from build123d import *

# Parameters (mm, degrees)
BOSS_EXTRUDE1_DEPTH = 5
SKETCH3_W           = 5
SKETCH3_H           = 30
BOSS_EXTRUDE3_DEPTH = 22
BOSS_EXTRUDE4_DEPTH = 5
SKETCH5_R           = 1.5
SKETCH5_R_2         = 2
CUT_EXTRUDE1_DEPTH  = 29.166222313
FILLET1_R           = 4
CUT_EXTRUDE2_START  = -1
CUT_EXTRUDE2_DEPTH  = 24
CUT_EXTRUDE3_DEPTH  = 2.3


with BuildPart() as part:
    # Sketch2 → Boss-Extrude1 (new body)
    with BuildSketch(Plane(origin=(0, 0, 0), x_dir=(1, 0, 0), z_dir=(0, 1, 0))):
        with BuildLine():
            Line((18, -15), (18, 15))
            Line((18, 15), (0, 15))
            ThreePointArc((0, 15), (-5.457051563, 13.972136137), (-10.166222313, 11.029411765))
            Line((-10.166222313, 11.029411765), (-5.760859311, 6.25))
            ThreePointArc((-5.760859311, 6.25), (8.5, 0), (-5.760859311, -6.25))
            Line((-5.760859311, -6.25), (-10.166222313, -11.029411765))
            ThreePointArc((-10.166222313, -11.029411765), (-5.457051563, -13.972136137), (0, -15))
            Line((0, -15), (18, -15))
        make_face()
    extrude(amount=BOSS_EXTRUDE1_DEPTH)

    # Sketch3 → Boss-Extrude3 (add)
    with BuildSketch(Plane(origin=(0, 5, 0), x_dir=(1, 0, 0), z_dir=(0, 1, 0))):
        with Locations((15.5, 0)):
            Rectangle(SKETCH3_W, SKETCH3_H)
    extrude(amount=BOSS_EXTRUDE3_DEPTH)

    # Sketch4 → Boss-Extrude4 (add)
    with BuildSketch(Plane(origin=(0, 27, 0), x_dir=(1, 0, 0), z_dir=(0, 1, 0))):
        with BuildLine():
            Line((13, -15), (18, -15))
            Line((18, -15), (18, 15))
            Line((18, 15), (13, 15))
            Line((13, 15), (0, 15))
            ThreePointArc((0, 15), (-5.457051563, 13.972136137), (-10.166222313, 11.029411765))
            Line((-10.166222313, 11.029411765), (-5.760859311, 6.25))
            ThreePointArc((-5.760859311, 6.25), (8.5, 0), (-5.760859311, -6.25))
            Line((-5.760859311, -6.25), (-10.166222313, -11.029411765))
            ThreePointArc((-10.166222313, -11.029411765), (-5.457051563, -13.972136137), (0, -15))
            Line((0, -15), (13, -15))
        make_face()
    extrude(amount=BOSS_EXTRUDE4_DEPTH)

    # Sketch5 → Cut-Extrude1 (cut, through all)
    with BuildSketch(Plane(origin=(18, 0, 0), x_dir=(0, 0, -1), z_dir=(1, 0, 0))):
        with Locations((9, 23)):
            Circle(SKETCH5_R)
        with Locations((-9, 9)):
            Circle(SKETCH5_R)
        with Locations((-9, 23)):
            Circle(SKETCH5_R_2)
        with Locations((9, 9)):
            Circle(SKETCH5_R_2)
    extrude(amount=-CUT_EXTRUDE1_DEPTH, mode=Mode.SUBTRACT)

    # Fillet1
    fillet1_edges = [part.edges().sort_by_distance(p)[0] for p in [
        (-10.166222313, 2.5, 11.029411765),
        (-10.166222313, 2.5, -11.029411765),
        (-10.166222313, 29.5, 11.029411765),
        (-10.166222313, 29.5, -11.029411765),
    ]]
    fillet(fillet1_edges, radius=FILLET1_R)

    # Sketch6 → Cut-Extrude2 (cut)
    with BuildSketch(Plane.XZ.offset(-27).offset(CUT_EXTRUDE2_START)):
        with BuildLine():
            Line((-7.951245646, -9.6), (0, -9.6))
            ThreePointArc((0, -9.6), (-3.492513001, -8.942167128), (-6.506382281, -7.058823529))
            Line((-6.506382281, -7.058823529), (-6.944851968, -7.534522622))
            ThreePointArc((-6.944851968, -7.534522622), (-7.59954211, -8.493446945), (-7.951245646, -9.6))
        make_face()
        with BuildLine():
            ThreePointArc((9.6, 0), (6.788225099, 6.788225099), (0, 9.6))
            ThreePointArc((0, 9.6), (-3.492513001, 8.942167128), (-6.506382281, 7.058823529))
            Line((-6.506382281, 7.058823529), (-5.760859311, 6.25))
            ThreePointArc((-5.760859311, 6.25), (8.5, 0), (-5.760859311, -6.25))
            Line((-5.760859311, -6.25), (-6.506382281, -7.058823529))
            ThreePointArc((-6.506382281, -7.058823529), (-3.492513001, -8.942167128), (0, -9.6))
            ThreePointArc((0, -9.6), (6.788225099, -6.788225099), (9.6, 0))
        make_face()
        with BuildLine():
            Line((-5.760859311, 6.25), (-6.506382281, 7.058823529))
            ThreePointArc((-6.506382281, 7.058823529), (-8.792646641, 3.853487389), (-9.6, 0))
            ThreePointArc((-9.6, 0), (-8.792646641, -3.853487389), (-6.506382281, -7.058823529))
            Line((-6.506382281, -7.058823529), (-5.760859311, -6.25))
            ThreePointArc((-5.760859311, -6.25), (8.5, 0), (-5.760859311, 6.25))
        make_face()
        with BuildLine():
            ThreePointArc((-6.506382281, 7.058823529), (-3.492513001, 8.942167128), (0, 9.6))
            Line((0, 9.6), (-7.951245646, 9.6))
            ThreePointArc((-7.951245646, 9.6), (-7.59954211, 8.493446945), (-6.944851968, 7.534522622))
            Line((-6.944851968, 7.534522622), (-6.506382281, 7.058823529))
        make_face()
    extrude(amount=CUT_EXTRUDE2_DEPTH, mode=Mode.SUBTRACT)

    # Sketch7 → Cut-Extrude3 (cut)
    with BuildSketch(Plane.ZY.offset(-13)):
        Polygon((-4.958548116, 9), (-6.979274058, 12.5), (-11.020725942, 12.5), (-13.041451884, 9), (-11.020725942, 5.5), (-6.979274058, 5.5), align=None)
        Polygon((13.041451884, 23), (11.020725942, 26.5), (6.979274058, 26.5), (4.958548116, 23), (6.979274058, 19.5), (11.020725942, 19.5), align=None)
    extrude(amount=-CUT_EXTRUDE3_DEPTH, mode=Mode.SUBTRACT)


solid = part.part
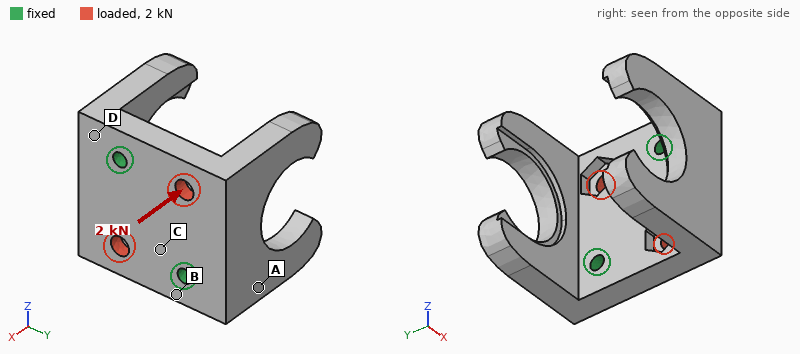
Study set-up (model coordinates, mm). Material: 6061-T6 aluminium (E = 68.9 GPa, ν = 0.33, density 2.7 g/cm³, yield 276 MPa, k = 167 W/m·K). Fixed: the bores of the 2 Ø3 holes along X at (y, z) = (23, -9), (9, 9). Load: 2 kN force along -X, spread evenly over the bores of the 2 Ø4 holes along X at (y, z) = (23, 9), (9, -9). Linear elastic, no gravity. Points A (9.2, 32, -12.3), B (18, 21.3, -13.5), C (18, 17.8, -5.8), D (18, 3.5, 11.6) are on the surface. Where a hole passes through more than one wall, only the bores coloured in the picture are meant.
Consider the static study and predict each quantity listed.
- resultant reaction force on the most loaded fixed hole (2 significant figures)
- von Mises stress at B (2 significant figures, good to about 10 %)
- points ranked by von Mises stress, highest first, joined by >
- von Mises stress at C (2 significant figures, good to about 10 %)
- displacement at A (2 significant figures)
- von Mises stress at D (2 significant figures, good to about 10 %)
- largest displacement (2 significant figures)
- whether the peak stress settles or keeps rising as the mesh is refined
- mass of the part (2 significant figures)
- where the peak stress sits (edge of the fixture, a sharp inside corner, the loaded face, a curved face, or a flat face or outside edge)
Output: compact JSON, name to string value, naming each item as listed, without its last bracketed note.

{"resultant reaction force on the most loaded fixed hole": "1.0 kN", "von Mises stress at B": "46 MPa", "points ranked by von Mises stress, highest first, joined by >": "C > B > D > A", "von Mises stress at C": "64 MPa", "displacement at A": "12 µm", "von Mises stress at D": "25 MPa", "largest displacement": "75 µm", "whether the peak stress settles or keeps rising as the mesh is refined": "keeps rising", "mass of the part": "22 g", "where the peak stress sits": "edge of the fixture"}
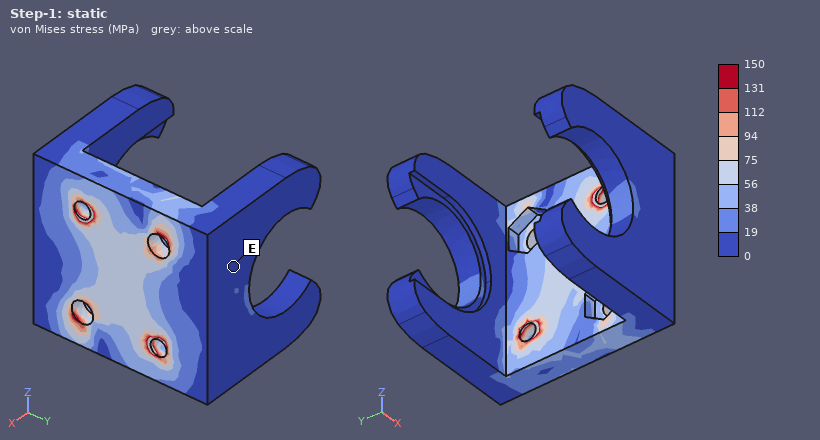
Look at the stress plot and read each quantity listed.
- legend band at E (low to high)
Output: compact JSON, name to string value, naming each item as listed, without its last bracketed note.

{"legend band at E": "0 to 19 MPa"}
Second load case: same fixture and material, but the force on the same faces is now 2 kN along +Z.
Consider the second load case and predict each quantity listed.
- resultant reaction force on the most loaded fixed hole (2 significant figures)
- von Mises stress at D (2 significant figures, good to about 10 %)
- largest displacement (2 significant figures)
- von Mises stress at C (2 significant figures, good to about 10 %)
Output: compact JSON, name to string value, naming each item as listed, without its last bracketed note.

{"resultant reaction force on the most loaded fixed hole": "1.0 kN", "von Mises stress at D": "6.9 MPa", "largest displacement": "12 µm", "von Mises stress at C": "13 MPa"}
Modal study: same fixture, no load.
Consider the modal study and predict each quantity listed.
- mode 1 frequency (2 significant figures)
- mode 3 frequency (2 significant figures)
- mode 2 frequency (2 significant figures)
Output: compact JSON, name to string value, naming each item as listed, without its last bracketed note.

{"mode 1 frequency": "5200 Hz", "mode 3 frequency": "7700 Hz", "mode 2 frequency": "5800 Hz"}
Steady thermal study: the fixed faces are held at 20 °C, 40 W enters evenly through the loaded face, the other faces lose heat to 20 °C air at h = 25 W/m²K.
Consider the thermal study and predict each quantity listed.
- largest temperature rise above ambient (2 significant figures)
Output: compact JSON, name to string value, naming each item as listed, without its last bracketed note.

{"largest temperature rise above ambient": "21 K"}
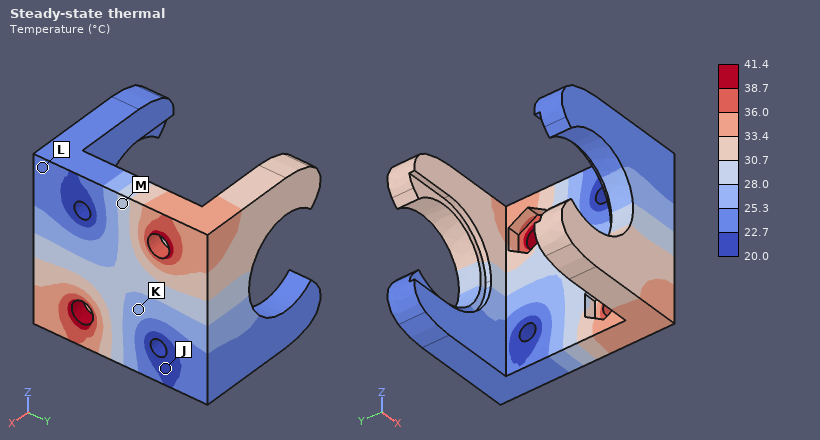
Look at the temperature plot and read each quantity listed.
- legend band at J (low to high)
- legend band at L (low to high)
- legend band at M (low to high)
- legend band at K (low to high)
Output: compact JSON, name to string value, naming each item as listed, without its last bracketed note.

{"legend band at J": "20.0 to 22.7 °C", "legend band at L": "22.7 to 25.3 °C", "legend band at M": "28.0 to 30.7 °C", "legend band at K": "25.3 to 28.0 °C"}
